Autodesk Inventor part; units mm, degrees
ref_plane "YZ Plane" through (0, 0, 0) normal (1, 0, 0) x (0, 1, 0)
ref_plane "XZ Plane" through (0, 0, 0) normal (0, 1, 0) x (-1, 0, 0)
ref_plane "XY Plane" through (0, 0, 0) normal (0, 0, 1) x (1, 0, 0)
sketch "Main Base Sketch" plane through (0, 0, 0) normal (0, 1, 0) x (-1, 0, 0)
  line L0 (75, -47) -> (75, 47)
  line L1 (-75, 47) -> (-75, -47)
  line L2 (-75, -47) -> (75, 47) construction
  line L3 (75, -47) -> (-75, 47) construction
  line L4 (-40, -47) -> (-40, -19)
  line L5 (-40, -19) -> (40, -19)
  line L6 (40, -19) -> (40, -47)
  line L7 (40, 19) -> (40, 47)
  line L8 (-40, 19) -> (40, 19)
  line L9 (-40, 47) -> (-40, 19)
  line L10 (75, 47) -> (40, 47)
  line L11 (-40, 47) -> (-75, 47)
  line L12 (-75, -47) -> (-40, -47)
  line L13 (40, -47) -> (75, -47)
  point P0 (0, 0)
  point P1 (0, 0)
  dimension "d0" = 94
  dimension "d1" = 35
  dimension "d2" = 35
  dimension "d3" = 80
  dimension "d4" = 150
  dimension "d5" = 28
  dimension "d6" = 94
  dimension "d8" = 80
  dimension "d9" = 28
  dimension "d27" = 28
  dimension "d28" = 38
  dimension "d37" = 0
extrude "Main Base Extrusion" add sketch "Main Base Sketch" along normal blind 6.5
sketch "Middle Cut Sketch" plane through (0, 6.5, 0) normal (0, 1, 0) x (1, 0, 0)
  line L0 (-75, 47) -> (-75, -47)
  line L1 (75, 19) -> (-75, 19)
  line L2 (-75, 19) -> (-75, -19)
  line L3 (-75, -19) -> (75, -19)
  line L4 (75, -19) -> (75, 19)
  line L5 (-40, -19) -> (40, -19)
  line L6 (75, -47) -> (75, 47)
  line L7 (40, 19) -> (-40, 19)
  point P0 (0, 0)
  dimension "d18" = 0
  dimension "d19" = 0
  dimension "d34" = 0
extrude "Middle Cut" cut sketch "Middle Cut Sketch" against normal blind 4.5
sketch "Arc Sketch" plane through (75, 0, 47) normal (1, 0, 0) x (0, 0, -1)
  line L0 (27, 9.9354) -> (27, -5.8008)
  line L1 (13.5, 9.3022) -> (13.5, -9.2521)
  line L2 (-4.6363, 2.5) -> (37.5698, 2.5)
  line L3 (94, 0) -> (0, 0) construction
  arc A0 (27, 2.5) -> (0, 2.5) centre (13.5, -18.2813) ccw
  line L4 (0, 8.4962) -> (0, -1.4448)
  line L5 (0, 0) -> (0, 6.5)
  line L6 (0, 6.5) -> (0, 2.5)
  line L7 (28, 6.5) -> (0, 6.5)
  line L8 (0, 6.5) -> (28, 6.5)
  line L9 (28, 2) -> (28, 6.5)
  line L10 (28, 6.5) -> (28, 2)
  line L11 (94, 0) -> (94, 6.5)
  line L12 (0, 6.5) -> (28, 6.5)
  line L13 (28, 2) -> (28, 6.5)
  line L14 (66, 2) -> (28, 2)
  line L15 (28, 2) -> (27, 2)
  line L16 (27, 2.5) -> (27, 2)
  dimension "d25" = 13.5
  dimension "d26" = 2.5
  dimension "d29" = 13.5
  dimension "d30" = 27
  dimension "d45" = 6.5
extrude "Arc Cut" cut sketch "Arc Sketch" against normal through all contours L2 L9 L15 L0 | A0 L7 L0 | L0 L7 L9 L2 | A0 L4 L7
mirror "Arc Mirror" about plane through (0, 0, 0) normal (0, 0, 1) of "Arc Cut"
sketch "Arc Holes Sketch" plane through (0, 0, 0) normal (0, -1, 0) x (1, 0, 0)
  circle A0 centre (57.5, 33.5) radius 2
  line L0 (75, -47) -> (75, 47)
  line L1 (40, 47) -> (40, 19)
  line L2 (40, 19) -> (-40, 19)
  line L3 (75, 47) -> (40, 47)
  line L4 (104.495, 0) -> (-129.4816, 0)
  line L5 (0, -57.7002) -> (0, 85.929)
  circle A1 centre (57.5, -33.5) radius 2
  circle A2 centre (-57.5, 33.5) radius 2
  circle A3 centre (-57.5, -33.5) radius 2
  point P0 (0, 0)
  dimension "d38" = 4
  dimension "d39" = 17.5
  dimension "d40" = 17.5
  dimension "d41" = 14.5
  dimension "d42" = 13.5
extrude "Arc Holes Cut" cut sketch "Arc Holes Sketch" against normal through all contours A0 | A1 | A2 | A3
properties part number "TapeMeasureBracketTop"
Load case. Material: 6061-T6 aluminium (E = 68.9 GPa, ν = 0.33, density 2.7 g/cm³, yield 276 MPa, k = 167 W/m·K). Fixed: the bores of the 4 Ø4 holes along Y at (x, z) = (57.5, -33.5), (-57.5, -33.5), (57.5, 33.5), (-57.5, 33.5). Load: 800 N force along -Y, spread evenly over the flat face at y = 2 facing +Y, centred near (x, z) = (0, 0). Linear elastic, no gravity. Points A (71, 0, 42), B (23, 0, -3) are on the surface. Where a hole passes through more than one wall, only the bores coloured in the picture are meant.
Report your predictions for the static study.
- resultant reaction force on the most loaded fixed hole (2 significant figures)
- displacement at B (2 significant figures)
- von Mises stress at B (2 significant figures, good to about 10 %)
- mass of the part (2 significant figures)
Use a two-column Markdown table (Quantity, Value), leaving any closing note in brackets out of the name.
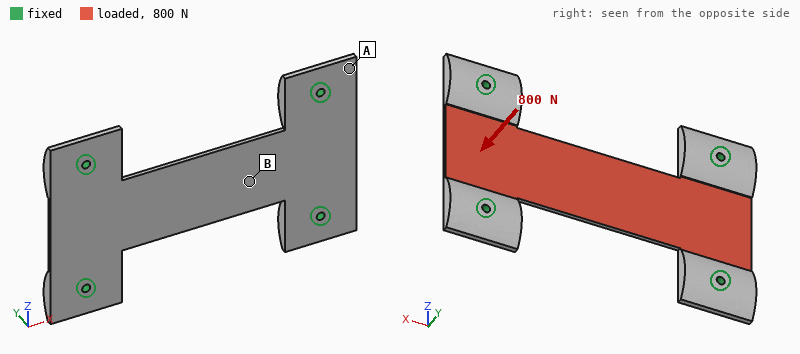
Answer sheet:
| Quantity | Value |
|---|---|
| resultant reaction force on the most loaded fixed hole | 410 N |
| displacement at B | 0.45 mm |
| von Mises stress at B | 29 MPa |
| mass of the part | 84 g |
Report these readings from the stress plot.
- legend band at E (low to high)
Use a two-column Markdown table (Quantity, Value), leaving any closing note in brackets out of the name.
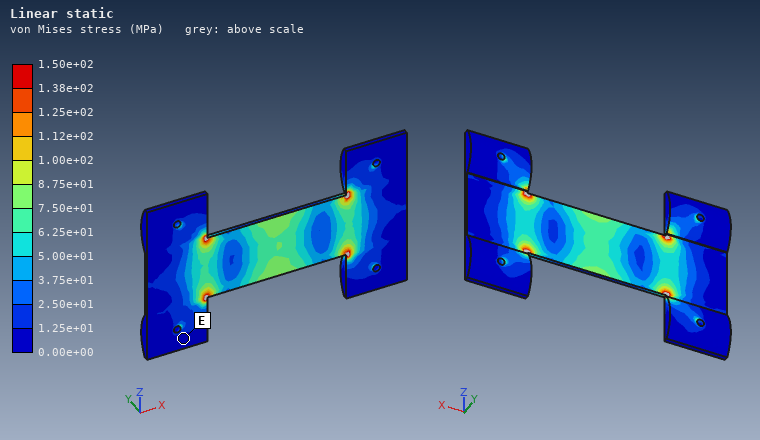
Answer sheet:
| Quantity | Value |
|---|---|
| legend band at E | 0.00e+00 to 1.25e+01 MPa |
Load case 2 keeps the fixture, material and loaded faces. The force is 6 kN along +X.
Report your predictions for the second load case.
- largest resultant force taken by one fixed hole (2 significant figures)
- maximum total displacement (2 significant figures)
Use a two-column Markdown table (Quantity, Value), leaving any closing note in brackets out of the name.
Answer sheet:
| Quantity | Value |
|---|---|
| largest resultant force taken by one fixed hole | 1.5 kN |
| maximum total displacement | 41 µm |
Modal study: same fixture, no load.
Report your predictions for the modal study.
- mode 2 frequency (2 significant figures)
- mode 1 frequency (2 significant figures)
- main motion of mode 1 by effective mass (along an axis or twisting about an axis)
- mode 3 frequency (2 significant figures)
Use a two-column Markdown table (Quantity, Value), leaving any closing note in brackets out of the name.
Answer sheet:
| Quantity | Value |
|---|---|
| mode 2 frequency | 2300 Hz |
| mode 1 frequency | 1100 Hz |
| main motion of mode 1 by effective mass | along Y |
| mode 3 frequency | 2800 Hz |
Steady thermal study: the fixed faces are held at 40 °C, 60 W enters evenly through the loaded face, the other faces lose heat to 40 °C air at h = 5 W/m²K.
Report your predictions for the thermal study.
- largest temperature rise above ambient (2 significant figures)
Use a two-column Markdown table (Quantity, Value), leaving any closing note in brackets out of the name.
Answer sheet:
| Quantity | Value |
|---|---|
| largest temperature rise above ambient | 52 K |
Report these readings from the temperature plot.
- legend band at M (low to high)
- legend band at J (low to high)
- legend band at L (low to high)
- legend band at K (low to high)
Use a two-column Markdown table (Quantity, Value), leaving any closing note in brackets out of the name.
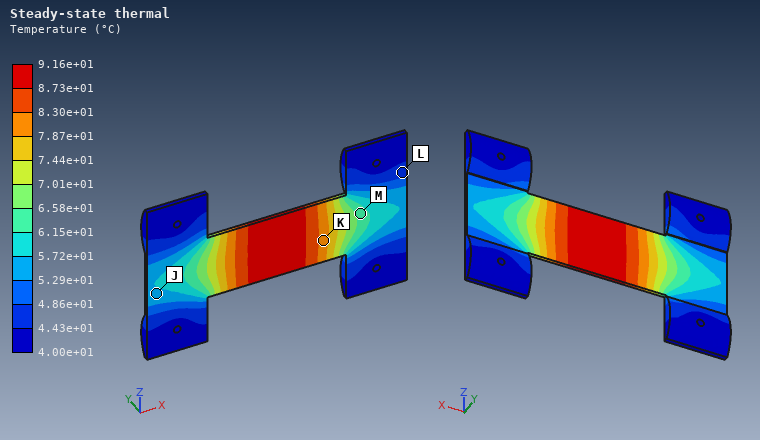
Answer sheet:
| Quantity | Value |
|---|---|
| legend band at M | 6.15e+01 to 6.58e+01 °C |
| legend band at J | 5.29e+01 to 5.72e+01 °C |
| legend band at L | 4.43e+01 to 4.86e+01 °C |
| legend band at K | 7.87e+01 to 8.30e+01 °C |
